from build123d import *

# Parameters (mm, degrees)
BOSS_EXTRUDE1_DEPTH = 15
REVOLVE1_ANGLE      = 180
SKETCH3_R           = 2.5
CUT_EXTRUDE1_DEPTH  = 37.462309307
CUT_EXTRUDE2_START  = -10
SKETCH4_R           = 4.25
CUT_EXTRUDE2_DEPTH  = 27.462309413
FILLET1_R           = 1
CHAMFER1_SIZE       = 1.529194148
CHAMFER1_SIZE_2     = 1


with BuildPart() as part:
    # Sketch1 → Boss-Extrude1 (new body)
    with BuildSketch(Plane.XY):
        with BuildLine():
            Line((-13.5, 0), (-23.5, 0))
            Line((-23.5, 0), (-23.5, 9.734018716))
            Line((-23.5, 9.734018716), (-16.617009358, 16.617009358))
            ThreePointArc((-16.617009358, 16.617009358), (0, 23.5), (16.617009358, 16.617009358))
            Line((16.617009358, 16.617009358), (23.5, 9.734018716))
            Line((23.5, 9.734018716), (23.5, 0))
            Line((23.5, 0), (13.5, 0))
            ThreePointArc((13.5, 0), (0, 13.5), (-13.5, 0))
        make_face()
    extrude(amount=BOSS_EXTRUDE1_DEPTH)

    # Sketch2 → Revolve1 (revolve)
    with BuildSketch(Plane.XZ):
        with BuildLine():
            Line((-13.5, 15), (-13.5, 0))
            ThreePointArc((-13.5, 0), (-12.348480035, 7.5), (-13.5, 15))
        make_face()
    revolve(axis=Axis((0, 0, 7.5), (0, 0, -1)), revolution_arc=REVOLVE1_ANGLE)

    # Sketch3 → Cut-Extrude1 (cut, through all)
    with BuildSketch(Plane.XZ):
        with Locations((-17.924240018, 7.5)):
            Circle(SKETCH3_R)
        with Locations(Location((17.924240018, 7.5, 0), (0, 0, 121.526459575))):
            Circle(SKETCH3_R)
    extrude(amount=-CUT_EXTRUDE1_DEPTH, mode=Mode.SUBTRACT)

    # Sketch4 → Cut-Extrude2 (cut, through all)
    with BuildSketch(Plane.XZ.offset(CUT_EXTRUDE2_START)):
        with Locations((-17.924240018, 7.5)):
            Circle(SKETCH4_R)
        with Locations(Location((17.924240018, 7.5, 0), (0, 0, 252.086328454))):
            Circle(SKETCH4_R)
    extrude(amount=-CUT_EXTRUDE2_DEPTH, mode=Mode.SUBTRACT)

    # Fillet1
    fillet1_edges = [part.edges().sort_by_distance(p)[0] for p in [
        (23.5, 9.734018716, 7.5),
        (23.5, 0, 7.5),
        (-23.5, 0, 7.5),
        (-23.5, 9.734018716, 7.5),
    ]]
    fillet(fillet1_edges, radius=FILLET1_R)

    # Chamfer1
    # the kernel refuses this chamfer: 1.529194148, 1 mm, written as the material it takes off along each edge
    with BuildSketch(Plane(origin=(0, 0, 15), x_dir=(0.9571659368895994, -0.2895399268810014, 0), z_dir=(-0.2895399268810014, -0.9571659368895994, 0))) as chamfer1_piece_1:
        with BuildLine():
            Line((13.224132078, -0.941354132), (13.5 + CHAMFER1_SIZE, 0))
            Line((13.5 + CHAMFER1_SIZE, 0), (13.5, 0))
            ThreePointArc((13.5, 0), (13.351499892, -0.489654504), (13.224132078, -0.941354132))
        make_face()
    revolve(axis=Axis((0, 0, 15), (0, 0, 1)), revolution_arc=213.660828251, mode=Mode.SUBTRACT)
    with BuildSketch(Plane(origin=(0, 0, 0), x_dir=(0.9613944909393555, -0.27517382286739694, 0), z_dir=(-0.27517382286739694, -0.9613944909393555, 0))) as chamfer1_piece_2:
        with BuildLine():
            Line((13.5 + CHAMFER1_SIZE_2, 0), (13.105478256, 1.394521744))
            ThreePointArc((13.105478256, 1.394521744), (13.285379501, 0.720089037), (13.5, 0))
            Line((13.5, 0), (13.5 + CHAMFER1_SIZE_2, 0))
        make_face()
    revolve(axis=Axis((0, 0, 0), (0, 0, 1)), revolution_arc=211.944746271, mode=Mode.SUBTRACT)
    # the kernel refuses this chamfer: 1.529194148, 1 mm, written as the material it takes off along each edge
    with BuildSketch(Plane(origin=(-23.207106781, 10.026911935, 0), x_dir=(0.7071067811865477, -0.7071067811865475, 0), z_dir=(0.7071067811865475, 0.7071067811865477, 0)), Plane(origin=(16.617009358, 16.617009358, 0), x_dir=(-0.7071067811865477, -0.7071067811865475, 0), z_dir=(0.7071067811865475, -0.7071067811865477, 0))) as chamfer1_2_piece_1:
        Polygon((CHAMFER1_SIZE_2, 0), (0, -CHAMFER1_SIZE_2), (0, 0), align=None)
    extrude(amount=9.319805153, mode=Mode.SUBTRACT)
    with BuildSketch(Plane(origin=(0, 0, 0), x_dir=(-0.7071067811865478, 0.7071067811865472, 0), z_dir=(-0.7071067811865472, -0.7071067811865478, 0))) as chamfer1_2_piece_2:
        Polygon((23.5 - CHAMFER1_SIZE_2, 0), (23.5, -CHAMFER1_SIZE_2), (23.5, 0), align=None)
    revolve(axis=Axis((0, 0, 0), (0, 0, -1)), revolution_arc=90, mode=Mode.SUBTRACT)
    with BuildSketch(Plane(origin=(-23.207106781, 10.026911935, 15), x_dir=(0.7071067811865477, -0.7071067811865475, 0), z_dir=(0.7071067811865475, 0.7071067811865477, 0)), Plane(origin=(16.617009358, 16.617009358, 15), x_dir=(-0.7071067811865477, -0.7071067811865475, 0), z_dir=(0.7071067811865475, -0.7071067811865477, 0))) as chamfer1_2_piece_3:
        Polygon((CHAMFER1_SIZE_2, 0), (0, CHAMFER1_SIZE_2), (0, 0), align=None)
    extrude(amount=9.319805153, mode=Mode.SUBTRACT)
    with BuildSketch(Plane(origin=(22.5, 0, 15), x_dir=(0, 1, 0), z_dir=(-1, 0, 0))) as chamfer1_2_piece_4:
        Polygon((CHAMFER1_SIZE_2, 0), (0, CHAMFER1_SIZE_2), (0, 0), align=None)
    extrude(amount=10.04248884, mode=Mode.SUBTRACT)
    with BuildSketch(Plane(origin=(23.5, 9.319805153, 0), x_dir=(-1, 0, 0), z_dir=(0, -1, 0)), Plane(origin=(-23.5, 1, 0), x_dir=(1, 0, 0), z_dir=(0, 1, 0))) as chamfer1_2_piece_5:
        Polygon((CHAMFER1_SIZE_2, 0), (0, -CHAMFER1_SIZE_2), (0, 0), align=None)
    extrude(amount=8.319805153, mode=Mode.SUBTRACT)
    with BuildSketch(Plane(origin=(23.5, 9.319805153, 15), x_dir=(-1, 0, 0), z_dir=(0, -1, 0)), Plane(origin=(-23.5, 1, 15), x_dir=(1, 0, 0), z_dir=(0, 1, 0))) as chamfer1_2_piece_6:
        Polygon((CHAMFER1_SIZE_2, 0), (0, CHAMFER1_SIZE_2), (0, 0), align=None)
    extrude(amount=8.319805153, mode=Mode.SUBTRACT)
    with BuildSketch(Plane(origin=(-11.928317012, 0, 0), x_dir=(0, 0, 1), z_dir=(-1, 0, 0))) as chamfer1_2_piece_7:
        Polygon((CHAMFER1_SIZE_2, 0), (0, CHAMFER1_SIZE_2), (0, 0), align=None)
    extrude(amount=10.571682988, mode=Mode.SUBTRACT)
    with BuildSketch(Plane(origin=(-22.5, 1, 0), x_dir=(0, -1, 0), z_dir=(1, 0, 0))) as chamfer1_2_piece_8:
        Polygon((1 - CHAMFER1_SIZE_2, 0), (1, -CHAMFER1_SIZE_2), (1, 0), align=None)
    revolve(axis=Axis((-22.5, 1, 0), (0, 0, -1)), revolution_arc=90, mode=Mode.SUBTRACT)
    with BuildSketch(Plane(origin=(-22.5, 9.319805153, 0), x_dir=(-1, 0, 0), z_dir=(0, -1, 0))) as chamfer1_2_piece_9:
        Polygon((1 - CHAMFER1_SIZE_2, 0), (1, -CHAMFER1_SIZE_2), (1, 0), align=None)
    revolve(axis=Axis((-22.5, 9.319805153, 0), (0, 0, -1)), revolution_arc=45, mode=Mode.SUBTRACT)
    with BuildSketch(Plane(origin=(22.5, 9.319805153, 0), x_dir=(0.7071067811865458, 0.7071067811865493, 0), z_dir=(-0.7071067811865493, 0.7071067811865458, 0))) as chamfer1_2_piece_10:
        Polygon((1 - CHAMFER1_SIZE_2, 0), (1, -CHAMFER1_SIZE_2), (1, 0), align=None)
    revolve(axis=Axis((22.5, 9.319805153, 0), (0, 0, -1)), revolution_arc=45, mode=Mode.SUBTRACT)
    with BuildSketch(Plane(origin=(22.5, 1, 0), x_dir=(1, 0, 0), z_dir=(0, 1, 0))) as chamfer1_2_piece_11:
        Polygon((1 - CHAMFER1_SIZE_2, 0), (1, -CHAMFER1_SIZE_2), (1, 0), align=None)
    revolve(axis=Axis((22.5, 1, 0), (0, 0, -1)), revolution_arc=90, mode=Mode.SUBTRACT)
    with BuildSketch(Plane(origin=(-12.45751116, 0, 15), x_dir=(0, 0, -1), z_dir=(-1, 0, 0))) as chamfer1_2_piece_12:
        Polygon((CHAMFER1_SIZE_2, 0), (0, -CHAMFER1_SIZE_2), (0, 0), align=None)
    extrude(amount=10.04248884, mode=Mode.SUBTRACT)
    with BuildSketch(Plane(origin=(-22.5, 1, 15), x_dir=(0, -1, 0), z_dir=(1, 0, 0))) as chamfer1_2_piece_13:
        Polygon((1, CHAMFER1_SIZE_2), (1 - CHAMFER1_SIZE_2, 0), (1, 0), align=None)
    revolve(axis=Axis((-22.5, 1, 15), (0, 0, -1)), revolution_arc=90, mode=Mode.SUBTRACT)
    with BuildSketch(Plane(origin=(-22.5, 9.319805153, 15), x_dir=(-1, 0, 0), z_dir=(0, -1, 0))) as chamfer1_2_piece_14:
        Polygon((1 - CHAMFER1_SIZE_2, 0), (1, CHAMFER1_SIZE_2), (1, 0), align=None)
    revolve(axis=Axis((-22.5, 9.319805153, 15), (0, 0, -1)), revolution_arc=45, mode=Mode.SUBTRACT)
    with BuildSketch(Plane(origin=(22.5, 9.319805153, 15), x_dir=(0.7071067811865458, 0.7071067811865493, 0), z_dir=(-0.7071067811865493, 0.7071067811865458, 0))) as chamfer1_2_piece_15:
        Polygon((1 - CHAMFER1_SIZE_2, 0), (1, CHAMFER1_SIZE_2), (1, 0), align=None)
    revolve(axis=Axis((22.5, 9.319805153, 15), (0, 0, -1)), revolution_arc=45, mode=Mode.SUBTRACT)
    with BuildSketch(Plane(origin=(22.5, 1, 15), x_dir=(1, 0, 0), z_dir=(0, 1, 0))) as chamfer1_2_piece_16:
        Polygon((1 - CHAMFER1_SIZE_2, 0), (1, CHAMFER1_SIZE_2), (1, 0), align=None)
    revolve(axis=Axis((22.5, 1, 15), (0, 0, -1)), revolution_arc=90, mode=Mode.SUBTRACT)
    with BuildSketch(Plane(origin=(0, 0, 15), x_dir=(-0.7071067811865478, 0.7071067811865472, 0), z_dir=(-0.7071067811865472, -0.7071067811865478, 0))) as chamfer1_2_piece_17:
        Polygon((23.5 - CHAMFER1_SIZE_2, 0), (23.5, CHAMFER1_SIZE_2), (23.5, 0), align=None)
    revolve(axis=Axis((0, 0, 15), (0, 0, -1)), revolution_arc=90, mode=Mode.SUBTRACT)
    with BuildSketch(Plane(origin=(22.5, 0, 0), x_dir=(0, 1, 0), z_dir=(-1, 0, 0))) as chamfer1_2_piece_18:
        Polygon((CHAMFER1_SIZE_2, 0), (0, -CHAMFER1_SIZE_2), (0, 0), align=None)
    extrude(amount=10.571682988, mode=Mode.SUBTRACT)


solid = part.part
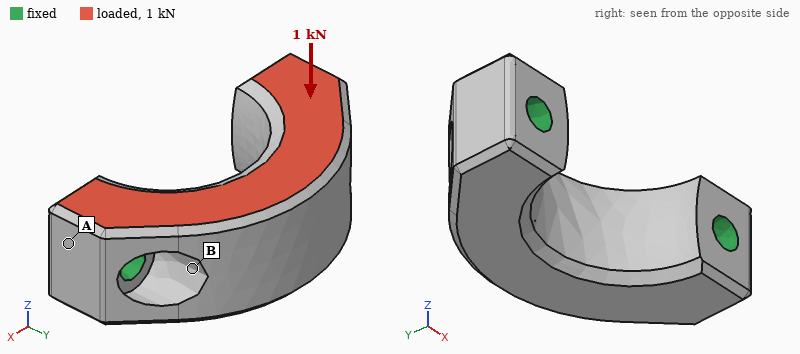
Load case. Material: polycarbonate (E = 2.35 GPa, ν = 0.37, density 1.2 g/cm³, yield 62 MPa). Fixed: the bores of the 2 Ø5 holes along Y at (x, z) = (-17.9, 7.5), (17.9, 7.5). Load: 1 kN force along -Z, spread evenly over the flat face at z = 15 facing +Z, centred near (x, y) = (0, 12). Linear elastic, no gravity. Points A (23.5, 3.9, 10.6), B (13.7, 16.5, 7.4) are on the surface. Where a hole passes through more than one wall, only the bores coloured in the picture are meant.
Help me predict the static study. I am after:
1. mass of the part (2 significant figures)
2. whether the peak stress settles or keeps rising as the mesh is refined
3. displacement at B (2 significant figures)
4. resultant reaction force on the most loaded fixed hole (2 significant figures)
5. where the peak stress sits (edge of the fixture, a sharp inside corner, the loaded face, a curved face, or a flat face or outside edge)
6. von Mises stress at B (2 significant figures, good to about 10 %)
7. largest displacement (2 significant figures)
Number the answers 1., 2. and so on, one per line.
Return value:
1. 10 g
2. keeps rising
3. 0.11 mm
4. 500 N
5. edge of the fixture
6. 8.1 MPa
7. 0.21 mm
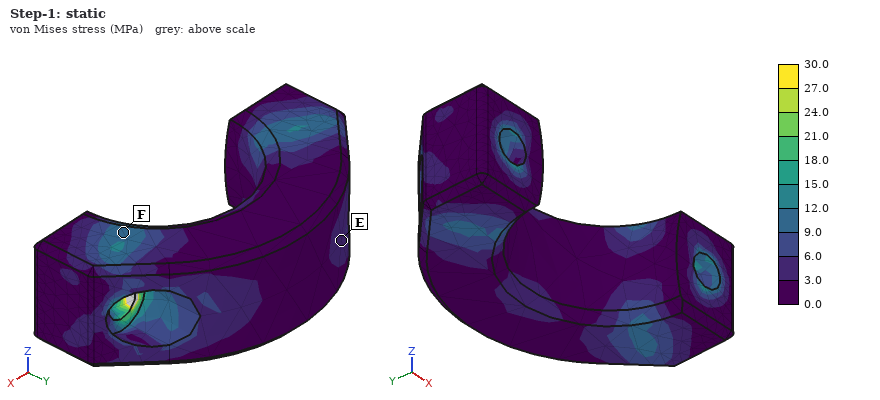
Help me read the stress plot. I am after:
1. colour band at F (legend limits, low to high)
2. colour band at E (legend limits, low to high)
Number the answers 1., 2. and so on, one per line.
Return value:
1. 9.0 to 12.0 MPa
2. 3.0 to 6.0 MPa
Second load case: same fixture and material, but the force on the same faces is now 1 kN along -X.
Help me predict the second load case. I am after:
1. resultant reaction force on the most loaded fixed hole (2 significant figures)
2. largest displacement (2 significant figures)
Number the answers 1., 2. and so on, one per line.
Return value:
1. 540 N
2. 76 µm
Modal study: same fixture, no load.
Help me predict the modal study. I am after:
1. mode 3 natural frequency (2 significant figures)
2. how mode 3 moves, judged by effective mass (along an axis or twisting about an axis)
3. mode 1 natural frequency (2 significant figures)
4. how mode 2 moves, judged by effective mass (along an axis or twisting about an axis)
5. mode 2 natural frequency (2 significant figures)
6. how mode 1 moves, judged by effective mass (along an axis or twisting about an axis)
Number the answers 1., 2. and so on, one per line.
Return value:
1. 9500 Hz
2. along Y
3. 4200 Hz
4. along X
5. 9100 Hz
6. along Z
